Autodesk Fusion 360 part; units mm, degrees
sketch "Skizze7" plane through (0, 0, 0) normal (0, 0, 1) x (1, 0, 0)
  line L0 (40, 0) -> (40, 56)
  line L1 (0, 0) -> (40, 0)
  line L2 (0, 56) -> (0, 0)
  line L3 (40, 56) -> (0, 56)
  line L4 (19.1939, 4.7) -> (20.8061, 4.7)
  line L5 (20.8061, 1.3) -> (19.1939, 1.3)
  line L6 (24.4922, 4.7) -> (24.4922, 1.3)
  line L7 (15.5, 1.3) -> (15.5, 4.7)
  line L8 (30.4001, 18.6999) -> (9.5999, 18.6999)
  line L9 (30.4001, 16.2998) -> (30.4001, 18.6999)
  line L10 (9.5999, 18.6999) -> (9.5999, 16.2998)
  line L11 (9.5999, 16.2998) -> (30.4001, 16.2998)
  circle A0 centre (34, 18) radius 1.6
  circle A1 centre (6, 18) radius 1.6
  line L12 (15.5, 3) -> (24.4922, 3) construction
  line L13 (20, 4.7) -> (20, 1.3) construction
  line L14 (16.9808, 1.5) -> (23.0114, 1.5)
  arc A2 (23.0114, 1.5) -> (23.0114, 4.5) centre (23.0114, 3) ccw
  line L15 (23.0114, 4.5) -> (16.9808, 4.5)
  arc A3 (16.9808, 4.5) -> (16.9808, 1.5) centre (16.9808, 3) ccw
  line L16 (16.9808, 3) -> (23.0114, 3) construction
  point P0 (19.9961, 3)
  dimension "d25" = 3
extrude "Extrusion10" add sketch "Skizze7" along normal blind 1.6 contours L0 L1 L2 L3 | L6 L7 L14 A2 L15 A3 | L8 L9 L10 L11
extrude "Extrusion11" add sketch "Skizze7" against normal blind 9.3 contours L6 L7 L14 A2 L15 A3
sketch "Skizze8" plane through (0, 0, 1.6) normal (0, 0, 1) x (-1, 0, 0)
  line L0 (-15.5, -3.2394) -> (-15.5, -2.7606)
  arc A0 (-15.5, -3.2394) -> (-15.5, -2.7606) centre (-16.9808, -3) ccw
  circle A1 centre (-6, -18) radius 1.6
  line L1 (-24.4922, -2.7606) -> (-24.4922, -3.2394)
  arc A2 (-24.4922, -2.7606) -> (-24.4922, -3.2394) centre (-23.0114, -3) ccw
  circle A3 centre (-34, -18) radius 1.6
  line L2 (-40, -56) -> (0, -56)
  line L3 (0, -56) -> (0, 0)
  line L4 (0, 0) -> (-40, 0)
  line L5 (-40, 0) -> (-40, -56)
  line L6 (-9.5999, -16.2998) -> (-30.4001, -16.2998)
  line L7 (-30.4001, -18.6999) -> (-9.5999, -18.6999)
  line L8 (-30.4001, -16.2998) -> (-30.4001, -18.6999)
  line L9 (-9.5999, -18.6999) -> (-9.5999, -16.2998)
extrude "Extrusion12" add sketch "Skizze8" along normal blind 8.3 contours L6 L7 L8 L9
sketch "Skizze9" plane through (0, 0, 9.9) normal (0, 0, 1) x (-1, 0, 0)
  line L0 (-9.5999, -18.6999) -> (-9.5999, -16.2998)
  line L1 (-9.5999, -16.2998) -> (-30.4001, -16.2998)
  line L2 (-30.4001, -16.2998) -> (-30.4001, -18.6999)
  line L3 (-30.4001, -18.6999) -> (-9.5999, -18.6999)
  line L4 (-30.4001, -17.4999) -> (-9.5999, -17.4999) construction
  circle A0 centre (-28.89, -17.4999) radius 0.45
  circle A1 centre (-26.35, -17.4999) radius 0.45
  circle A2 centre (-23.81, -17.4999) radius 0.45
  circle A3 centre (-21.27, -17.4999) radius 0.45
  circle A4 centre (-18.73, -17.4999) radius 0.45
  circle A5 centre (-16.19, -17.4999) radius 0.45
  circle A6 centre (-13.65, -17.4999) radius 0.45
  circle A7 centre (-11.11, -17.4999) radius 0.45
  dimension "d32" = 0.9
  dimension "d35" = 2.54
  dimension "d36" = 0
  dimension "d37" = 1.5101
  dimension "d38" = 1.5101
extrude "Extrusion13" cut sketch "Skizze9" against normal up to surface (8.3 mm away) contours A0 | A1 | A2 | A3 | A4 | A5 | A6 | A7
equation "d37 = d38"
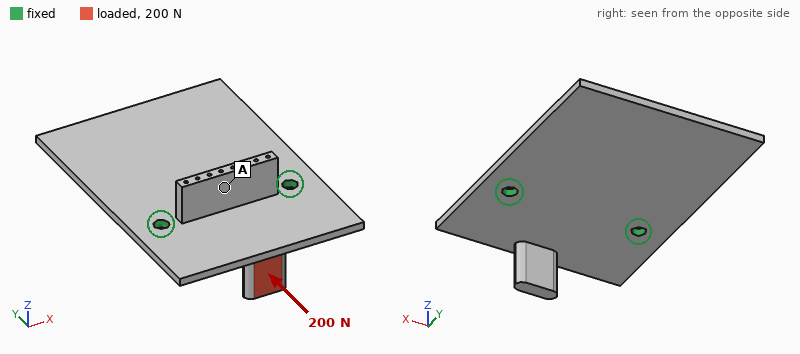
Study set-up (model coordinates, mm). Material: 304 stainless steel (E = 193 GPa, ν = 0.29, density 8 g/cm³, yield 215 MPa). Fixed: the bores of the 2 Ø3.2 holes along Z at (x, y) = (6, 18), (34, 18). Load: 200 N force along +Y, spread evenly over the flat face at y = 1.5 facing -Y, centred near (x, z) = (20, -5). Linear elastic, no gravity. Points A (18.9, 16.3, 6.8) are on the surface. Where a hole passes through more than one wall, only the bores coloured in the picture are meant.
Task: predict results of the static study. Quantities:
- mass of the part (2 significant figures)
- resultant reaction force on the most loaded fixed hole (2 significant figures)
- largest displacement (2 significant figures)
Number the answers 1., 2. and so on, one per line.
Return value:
1. 33 g
2. 100 N
3. 0.11 mm
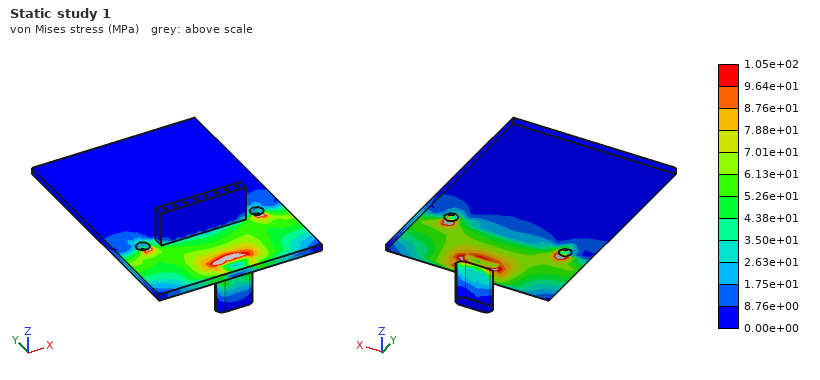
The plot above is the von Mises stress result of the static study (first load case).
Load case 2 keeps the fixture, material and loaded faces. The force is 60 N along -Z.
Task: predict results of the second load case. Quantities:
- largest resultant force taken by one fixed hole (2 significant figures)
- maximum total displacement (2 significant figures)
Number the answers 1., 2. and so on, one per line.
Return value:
1. 33 N
2. 56 µm
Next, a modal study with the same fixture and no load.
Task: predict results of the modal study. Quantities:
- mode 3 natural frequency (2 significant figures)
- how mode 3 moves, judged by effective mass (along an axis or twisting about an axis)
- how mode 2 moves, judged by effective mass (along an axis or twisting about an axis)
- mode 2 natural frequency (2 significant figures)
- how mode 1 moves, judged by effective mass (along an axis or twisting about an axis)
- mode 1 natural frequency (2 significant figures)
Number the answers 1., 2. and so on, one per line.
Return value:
1. 2900 Hz
2. along Z
3. twisting about Y
4. 2200 Hz
5. along Z
6. 880 Hz
